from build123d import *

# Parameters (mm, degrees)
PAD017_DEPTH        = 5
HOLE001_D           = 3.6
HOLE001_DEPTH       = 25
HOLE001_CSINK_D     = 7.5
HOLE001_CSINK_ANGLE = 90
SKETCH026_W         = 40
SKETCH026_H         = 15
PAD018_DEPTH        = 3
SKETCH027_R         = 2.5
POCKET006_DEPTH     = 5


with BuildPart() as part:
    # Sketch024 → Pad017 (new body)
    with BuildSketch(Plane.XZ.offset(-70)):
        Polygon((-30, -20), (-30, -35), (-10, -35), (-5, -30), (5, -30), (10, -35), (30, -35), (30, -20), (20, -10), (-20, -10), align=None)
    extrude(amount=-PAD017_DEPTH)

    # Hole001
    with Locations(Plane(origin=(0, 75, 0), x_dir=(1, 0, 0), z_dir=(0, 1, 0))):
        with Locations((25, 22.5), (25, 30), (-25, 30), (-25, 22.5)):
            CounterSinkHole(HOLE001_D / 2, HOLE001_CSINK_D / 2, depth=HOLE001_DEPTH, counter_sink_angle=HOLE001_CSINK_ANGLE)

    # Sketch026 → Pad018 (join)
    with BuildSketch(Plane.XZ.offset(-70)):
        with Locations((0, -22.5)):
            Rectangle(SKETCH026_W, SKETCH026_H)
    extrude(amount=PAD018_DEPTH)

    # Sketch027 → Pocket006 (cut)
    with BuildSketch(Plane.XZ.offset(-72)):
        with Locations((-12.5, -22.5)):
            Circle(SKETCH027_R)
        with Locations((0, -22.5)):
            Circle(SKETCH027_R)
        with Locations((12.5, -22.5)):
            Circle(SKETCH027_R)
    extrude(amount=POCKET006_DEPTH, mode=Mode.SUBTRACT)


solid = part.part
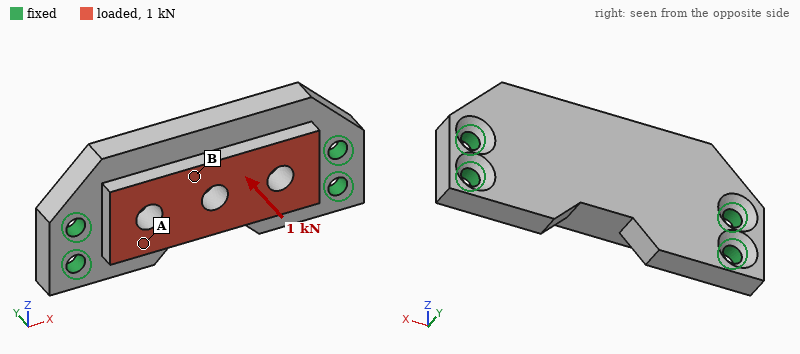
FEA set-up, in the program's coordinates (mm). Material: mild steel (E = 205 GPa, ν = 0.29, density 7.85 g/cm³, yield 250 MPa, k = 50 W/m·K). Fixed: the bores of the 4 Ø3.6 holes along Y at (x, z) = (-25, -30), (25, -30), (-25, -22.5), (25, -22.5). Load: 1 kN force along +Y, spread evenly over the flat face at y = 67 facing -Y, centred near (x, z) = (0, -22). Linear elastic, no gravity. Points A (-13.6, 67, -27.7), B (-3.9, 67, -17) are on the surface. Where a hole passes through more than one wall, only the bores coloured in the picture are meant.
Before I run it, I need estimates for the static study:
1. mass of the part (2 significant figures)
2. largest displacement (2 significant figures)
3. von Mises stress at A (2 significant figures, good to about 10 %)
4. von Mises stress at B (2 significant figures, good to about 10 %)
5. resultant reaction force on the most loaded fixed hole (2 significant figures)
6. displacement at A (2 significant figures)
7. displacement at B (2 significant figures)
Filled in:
61 g
9.8 µm
12 MPa
29 MPa
410 N
4.3 µm
8.2 µm
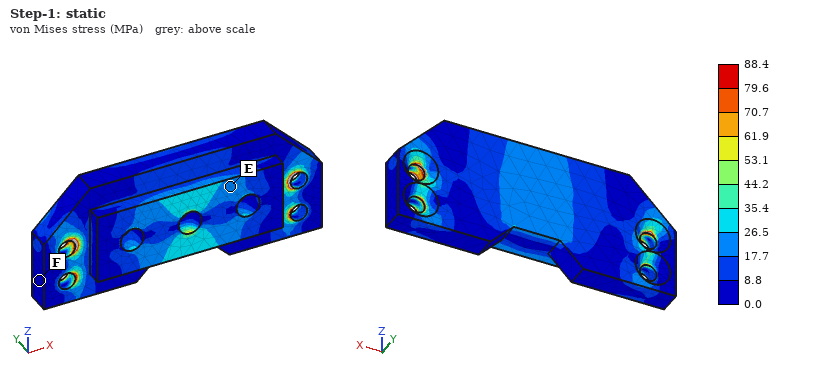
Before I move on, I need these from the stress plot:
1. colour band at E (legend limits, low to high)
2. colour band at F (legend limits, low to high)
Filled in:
17.7 to 26.5 MPa
0.0 to 8.8 MPa
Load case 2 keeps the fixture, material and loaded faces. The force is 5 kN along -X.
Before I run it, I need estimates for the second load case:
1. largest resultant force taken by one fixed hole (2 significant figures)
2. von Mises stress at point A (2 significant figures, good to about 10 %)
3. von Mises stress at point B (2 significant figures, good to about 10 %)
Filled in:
1.6 kN
21 MPa
16 MPa
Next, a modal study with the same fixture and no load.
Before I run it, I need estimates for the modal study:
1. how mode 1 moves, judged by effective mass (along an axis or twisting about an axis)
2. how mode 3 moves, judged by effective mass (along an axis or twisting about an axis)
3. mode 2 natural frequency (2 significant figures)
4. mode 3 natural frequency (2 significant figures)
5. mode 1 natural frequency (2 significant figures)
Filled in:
along Y
along Z
15 kHz
20 kHz
8600 Hz
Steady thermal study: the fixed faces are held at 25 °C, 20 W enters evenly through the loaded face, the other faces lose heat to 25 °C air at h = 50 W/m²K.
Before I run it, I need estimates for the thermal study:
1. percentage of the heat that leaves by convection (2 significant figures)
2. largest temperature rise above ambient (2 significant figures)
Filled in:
12 %
26 K
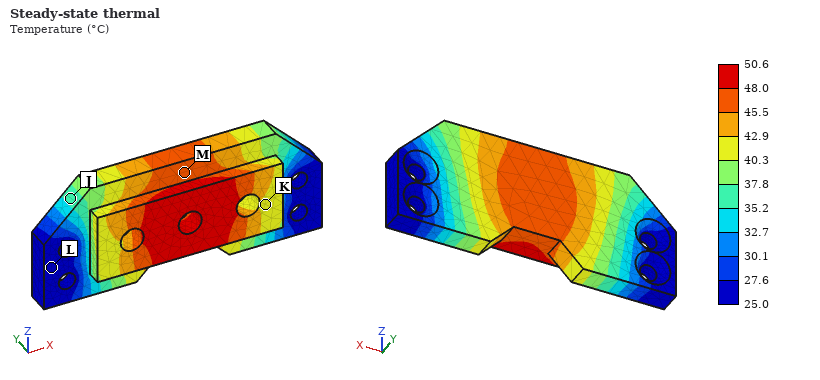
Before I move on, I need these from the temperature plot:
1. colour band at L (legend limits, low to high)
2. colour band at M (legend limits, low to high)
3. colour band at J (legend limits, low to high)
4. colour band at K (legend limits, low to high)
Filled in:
25.0 to 27.6 °C
45.5 to 48.0 °C
35.2 to 37.8 °C
40.3 to 42.9 °C
